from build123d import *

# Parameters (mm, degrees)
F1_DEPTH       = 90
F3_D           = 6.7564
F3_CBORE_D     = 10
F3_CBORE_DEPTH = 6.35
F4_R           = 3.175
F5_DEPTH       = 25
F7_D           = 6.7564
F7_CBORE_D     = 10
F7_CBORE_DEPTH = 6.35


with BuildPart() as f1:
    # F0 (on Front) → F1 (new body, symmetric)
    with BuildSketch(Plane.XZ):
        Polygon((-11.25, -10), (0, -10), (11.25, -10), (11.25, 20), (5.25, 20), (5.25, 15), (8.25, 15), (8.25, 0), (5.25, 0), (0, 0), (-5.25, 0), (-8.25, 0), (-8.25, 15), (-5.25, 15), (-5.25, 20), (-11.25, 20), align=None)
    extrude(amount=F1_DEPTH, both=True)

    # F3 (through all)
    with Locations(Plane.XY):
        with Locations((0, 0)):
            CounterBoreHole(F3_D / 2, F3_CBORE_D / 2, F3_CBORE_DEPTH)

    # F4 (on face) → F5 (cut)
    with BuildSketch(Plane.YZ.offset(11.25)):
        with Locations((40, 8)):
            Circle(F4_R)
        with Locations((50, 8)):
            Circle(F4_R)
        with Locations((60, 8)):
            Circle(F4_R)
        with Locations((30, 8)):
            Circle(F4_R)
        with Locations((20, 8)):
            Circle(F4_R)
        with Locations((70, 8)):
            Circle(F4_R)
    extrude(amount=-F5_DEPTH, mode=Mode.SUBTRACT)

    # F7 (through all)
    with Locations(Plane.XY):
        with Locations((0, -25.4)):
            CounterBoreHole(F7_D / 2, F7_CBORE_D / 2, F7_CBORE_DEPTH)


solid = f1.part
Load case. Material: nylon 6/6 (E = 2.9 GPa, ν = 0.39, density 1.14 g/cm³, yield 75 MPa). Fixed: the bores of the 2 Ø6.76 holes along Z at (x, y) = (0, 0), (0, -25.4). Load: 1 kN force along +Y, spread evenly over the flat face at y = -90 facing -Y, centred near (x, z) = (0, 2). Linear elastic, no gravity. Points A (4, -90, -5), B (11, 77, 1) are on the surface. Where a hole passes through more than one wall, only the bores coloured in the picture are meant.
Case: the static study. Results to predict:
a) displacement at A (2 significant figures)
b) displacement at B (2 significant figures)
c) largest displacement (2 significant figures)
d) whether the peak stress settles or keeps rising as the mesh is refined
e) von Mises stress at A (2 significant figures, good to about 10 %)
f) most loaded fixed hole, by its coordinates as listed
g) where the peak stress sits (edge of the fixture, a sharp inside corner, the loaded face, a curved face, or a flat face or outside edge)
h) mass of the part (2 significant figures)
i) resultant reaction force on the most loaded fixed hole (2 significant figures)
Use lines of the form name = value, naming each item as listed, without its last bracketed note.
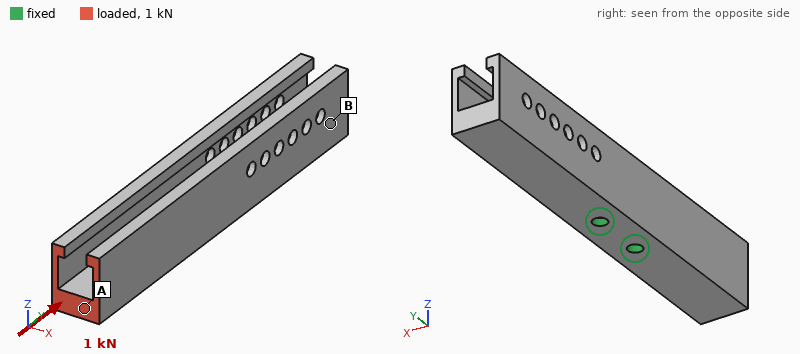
displacement at A = 0.25 mm
displacement at B = 0.24 mm
largest displacement = 0.29 mm
whether the peak stress settles or keeps rising as the mesh is refined = keeps rising
von Mises stress at A = 2.7 MPa
most loaded fixed hole, by its coordinates as listed = (0, -25.4)
where the peak stress sits = edge of the fixture
mass of the part = 74 g
resultant reaction force on the most loaded fixed hole = 740 N
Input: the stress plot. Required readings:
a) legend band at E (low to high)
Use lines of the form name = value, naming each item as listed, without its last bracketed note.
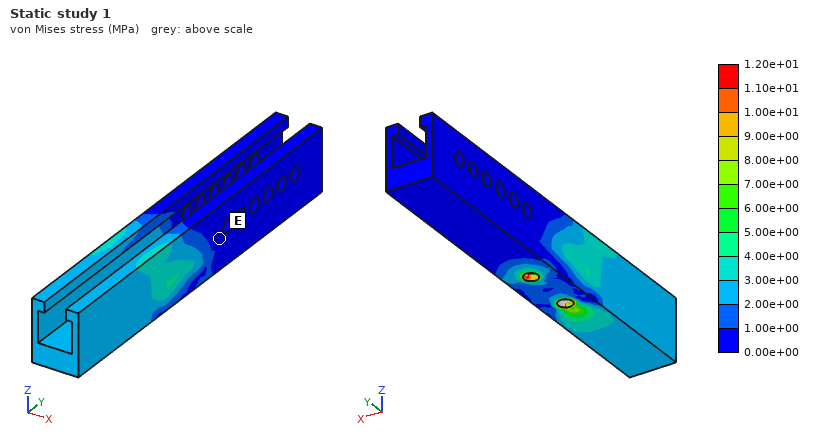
legend band at E = 0.00e+00 to 1.00e+00 MPa
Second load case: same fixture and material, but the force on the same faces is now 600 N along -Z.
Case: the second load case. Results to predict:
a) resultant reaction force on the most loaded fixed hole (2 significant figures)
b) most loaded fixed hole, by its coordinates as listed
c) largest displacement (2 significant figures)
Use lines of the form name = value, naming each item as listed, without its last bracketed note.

resultant reaction force on the most loaded fixed hole = 2.0 kN
most loaded fixed hole, by its coordinates as listed = (0, -25.4)
largest displacement = 2.0 mm
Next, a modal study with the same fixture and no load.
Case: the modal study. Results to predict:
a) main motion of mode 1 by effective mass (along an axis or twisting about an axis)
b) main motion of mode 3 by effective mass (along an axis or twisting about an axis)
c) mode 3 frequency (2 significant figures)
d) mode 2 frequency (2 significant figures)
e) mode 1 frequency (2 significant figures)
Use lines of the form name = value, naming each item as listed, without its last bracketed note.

main motion of mode 1 by effective mass = along X
main motion of mode 3 by effective mass = along X
mode 3 frequency = 670 Hz
mode 2 frequency = 540 Hz
mode 1 frequency = 450 Hz
